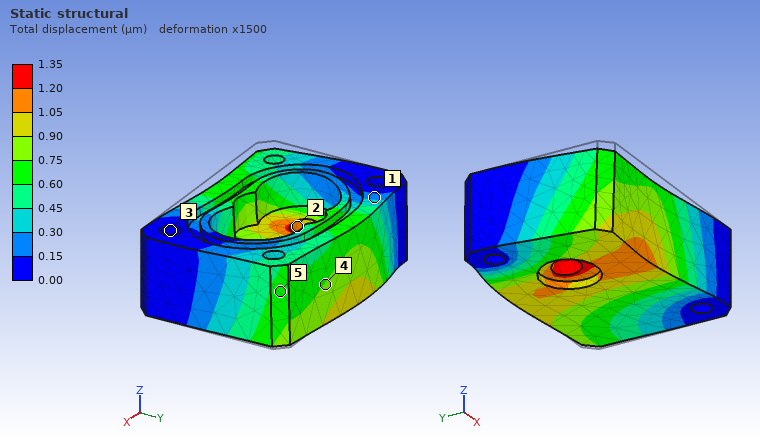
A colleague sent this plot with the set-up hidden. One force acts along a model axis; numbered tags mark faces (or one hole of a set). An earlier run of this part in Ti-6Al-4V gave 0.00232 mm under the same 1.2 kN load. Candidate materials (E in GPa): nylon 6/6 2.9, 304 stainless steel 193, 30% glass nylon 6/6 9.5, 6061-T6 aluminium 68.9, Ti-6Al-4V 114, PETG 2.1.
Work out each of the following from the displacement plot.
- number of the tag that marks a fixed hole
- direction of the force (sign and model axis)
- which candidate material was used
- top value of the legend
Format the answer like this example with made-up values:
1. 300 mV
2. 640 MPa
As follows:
1. 3
2. +Y
3. 304 stainless steel
4. 1.35 µm
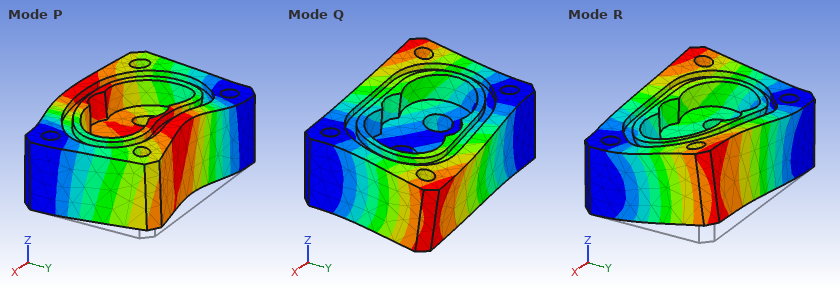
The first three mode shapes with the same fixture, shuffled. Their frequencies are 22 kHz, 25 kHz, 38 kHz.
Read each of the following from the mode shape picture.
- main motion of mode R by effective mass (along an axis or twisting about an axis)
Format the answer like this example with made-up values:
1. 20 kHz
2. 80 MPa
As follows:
1. along Z
